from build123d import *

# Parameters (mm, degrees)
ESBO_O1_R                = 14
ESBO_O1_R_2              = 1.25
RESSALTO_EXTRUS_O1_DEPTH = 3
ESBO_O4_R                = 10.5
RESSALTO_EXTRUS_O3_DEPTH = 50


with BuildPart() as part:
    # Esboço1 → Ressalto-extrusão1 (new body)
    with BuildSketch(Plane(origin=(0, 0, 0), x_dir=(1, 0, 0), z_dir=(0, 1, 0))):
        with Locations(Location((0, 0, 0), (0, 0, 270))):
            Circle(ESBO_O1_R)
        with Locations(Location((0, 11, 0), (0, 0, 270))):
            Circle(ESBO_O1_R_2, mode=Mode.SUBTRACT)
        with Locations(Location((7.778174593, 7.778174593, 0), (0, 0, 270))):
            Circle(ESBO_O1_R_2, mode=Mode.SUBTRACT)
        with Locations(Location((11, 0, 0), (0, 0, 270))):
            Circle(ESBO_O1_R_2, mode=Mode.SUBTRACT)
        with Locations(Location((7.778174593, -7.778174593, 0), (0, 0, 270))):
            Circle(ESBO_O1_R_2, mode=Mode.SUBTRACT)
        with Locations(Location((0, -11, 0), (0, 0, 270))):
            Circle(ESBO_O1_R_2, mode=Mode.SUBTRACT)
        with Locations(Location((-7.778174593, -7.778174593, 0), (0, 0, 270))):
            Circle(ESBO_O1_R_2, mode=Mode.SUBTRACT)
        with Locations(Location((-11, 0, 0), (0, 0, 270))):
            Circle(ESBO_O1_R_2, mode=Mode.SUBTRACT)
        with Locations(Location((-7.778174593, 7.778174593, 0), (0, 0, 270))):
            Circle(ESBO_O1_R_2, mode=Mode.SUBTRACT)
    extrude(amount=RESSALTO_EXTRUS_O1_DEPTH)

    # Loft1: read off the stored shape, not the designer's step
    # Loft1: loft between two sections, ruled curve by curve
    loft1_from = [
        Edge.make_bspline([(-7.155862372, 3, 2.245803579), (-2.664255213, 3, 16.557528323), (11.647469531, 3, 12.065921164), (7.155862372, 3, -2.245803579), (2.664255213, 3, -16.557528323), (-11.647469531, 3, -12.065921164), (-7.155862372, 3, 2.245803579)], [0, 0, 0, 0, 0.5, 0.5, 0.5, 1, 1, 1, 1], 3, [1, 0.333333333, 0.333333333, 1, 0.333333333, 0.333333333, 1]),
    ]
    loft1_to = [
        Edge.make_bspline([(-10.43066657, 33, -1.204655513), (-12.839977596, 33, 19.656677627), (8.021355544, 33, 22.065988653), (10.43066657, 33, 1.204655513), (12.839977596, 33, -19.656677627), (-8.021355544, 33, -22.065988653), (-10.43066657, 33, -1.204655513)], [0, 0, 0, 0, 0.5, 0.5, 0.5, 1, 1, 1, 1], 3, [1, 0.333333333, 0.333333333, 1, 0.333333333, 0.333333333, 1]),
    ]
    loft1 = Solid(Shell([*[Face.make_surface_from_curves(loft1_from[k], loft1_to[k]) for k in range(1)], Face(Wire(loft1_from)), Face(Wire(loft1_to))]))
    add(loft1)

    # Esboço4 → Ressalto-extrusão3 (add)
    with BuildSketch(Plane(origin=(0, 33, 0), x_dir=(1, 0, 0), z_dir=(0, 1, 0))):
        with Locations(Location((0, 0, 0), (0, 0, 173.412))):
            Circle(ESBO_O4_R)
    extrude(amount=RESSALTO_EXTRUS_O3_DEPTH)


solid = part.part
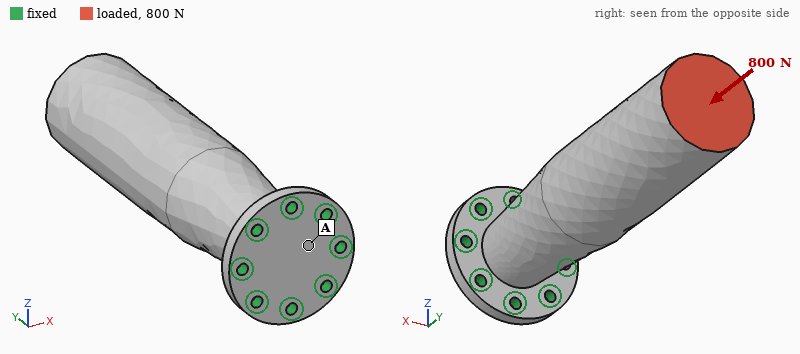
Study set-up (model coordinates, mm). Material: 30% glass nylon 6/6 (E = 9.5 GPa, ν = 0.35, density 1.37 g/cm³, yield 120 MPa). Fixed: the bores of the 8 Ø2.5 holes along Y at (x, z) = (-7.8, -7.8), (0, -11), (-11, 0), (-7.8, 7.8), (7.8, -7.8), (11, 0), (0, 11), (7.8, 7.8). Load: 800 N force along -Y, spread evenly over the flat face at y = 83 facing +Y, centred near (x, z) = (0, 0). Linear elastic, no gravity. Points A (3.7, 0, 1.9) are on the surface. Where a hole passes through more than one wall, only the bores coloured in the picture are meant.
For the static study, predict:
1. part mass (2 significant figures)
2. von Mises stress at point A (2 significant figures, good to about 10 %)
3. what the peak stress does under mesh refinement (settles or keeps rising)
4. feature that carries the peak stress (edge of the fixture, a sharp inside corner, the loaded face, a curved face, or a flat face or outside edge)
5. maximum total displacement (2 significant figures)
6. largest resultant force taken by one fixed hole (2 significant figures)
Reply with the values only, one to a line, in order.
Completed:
36 g
5.7 MPa
keeps rising
edge of the fixture
34 µm
110 N
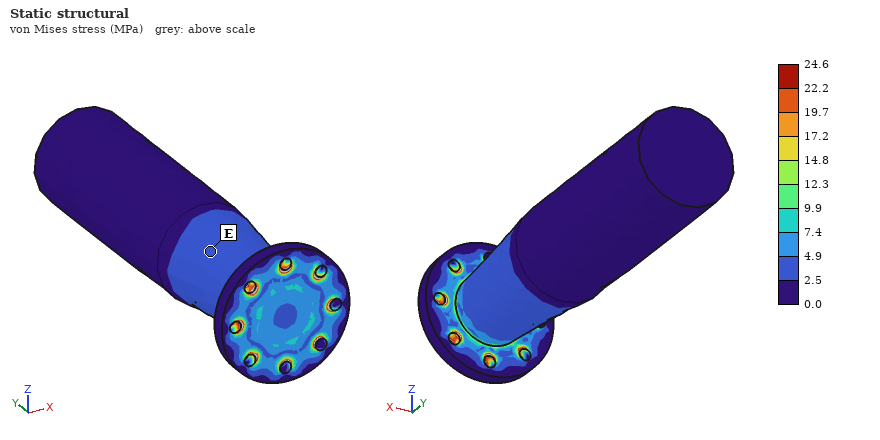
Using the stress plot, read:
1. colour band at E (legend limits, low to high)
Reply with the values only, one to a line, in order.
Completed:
2.5 to 4.9 MPa
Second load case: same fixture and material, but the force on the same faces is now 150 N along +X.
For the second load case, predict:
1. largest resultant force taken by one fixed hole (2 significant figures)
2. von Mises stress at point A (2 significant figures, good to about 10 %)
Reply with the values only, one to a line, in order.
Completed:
340 N
19 MPa
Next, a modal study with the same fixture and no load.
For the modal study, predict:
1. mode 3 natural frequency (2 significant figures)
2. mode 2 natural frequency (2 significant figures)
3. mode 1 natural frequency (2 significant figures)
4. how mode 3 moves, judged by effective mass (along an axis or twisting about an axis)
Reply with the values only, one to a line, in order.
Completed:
3500 Hz
600 Hz
600 Hz
twisting about Y
